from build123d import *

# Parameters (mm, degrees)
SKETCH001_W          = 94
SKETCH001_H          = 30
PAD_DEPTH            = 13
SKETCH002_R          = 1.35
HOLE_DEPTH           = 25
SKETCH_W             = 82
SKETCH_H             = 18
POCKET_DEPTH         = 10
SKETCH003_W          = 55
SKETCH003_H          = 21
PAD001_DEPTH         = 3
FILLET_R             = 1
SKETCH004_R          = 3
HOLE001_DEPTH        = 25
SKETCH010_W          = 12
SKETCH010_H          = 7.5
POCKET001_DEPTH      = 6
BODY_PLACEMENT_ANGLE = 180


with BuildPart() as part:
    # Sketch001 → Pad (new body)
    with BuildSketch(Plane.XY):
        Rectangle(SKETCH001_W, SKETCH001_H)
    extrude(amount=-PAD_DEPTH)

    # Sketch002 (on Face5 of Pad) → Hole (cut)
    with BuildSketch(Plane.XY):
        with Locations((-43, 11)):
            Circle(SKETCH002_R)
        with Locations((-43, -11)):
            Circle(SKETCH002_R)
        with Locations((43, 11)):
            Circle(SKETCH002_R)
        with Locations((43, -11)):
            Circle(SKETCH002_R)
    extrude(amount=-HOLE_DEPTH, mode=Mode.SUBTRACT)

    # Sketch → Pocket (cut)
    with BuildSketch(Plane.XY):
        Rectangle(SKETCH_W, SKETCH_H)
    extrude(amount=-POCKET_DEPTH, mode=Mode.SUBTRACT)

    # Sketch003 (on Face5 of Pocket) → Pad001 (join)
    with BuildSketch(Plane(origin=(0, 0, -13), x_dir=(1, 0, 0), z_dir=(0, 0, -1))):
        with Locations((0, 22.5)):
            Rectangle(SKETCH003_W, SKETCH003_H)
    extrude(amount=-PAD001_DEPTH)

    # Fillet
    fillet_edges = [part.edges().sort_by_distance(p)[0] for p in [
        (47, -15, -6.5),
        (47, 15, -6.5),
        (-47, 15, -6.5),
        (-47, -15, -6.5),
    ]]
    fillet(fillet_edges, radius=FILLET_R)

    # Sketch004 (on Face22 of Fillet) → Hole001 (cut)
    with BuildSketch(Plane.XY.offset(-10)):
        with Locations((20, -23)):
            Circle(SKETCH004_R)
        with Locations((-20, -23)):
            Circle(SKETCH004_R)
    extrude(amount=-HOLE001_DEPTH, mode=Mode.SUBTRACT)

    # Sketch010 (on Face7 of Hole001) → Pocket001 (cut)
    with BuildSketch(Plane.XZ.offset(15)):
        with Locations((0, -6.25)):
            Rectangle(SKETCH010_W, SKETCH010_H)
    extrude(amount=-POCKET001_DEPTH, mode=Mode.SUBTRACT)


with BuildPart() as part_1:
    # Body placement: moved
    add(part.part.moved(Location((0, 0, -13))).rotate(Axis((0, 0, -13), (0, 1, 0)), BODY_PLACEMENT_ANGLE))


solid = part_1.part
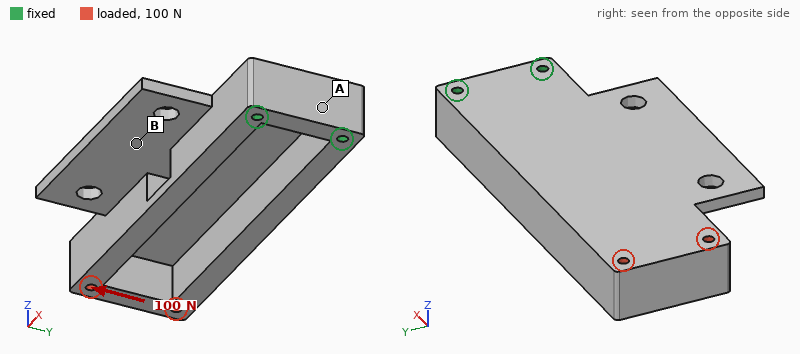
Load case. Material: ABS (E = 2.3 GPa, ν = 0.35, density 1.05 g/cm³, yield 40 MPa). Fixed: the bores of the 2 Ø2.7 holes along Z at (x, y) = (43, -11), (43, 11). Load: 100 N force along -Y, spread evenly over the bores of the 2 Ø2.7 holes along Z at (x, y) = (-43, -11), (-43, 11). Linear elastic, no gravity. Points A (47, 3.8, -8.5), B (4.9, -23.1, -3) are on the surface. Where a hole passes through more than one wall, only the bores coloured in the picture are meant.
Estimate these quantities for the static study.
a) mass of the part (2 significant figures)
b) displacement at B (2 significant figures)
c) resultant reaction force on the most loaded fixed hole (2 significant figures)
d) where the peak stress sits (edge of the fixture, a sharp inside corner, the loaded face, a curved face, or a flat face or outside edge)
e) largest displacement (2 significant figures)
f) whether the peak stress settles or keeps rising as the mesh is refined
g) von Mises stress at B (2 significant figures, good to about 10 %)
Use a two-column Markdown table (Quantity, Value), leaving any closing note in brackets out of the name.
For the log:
| Quantity | Value |
|---|---|
| mass of the part | 25 g |
| displacement at B | 0.40 mm |
| resultant reaction force on the most loaded fixed hole | 360 N |
| where the peak stress sits | edge of the fixture |
| largest displacement | 1.2 mm |
| whether the peak stress settles or keeps rising as the mesh is refined | keeps rising |
| von Mises stress at B | 1.7 MPa |
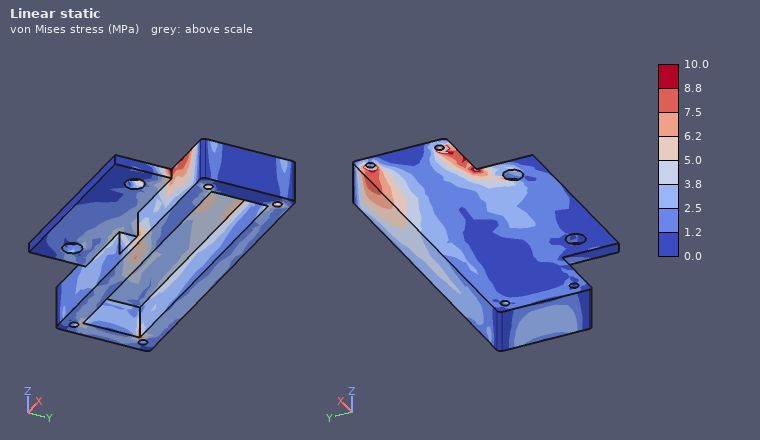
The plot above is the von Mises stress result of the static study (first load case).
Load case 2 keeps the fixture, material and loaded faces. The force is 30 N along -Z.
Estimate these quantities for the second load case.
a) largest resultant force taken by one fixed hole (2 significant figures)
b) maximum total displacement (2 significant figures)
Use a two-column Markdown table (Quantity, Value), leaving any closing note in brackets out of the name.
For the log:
| Quantity | Value |
|---|---|
| largest resultant force taken by one fixed hole | 21 N |
| maximum total displacement | 1.0 mm |
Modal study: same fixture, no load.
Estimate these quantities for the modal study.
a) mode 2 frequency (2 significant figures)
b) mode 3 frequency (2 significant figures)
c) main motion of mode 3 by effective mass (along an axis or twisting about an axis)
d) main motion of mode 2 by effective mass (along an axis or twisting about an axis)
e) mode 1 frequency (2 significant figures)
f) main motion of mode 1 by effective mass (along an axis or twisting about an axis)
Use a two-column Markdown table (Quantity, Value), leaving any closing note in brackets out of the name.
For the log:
| Quantity | Value |
|---|---|
| mode 2 frequency | 530 Hz |
| mode 3 frequency | 950 Hz |
| main motion of mode 3 by effective mass | along Y |
| main motion of mode 2 by effective mass | along Y |
| mode 1 frequency | 340 Hz |
| main motion of mode 1 by effective mass | along Z |
